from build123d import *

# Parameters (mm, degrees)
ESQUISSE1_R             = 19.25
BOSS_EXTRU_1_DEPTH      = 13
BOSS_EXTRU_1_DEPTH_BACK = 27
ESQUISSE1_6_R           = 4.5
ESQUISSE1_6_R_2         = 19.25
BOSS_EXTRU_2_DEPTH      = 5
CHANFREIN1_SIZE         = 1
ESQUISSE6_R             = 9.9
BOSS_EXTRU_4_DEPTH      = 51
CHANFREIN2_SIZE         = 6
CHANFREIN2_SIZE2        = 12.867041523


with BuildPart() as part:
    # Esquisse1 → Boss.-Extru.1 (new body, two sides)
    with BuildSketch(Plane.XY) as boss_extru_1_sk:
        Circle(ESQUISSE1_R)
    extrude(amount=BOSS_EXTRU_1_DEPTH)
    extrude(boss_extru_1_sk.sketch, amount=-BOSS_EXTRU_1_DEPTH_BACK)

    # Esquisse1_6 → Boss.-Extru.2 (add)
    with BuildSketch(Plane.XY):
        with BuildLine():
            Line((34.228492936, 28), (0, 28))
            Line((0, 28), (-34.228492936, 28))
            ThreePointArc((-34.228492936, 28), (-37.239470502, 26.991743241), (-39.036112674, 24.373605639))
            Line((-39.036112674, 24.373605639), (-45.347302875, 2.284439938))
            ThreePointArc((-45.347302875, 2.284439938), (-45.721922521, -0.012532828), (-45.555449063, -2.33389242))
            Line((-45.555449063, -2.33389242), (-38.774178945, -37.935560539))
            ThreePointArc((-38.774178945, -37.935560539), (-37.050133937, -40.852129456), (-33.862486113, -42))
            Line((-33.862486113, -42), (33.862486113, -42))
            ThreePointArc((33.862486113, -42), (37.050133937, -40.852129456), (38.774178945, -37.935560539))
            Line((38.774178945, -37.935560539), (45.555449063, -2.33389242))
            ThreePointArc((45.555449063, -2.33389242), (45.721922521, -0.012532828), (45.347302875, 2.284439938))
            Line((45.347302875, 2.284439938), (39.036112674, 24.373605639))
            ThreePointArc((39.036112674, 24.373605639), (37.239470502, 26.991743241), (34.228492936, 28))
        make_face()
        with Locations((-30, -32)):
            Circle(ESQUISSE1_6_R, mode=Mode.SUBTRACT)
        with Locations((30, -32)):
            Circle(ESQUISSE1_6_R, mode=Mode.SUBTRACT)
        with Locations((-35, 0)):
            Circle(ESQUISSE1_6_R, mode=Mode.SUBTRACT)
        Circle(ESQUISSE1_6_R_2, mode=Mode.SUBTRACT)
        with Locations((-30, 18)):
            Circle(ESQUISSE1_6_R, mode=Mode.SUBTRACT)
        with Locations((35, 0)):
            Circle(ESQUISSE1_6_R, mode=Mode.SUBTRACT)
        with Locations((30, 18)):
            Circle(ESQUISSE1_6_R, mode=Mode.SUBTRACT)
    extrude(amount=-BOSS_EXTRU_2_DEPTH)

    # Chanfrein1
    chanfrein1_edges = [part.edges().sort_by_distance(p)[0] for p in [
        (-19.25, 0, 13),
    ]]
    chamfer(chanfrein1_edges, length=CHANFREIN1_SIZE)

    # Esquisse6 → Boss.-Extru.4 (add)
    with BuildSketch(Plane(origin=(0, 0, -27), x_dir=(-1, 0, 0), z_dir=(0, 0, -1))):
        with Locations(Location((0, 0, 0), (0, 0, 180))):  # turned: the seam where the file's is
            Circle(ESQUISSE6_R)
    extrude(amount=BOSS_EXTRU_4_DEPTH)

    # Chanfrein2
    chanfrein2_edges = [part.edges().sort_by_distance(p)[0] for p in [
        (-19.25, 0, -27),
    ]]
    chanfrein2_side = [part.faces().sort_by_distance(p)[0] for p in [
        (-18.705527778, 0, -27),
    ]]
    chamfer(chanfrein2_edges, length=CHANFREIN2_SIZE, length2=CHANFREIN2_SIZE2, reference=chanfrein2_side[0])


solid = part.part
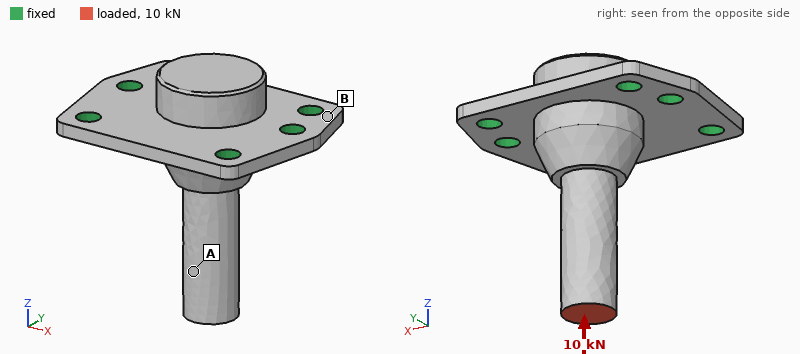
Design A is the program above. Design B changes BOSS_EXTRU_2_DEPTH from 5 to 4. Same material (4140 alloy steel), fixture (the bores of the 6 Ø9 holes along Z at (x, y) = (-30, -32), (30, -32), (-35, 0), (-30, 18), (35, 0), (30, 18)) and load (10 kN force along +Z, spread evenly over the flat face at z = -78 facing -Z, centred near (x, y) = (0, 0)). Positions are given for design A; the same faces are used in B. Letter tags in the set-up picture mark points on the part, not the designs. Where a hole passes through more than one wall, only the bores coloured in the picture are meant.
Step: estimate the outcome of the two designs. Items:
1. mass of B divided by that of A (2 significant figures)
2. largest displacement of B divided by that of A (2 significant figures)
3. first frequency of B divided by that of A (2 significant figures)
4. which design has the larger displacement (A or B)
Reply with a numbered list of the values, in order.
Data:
1. 0.95
2. 1.5
3. 0.80
4. B
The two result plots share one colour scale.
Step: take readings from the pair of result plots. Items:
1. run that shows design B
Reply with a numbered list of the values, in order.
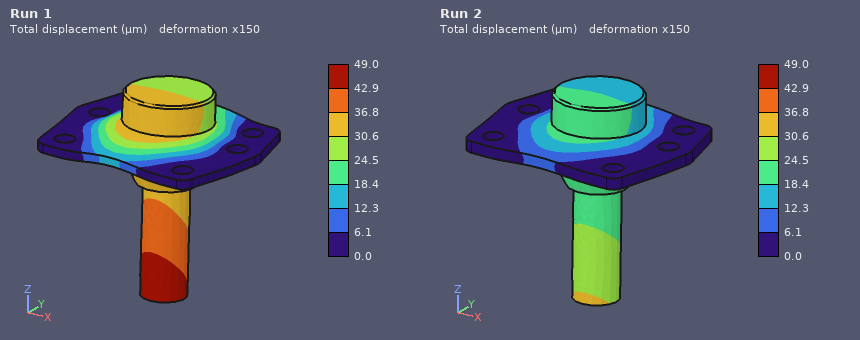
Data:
1. Run 1
